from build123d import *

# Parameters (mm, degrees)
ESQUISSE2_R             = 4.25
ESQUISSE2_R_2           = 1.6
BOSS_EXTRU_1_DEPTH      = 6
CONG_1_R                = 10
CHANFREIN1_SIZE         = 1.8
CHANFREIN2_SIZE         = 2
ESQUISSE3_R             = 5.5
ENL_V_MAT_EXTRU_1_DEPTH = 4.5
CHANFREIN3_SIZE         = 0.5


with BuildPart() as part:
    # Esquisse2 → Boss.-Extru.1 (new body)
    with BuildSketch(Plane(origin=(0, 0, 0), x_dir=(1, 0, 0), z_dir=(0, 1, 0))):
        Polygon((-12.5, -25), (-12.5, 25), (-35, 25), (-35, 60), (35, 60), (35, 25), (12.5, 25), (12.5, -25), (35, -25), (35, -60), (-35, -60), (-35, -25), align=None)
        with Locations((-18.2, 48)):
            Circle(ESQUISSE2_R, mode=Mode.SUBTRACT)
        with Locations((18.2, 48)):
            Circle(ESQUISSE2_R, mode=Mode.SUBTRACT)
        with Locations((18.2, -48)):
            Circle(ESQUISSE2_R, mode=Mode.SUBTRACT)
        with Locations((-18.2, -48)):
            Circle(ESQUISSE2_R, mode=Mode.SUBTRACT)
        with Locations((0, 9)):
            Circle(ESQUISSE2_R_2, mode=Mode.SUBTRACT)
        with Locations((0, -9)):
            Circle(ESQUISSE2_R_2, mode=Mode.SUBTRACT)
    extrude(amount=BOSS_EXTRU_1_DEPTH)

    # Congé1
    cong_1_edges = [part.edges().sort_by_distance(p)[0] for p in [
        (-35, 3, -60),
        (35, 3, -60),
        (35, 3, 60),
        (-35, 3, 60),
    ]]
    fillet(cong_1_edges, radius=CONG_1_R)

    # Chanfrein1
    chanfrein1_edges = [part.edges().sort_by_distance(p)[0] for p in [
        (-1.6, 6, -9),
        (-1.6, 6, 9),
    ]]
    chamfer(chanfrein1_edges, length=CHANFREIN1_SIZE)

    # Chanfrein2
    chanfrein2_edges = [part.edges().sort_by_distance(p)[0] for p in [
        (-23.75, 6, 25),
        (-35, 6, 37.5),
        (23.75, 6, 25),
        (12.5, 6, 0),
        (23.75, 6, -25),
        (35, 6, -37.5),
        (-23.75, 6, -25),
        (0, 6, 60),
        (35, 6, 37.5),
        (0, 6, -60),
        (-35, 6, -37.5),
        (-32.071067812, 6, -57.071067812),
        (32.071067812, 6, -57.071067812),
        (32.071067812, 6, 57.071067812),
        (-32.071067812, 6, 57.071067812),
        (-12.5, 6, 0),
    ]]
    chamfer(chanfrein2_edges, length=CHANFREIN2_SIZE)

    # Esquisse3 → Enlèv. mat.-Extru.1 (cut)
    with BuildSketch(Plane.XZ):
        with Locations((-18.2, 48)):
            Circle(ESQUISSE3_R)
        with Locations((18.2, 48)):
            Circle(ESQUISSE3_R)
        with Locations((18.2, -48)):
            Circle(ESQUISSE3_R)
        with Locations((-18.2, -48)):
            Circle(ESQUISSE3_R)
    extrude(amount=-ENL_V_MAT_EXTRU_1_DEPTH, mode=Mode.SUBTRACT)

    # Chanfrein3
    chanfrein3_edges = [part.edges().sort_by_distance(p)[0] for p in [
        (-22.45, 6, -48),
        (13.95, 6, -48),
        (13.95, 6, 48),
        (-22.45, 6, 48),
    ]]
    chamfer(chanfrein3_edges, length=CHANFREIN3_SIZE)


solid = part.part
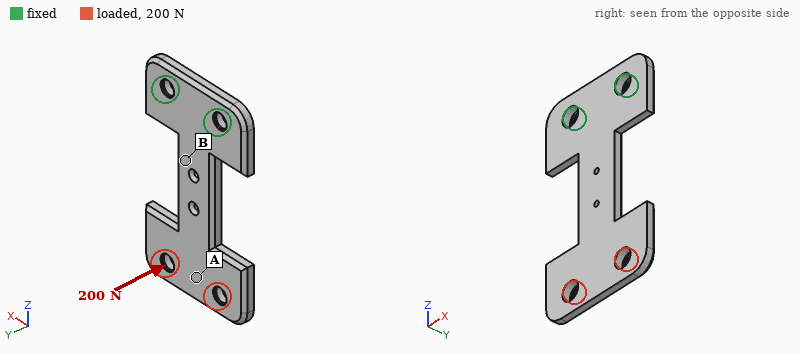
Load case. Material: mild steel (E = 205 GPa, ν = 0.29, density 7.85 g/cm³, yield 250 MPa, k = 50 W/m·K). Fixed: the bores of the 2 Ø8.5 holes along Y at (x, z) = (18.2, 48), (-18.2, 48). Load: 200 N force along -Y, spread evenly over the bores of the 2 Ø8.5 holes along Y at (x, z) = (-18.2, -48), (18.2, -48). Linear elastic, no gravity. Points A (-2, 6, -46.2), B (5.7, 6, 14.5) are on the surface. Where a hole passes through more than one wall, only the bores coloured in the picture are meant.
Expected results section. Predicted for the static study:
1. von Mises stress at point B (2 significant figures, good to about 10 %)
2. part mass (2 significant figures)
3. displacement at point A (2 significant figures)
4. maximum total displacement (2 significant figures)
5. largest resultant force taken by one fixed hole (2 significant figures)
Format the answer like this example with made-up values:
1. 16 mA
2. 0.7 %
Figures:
1. 96 MPa
2. 260 g
3. 0.64 mm
4. 0.78 mm
5. 270 N
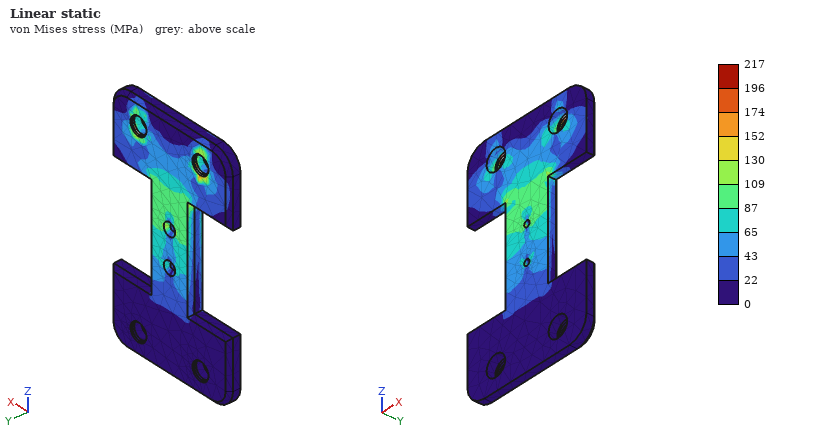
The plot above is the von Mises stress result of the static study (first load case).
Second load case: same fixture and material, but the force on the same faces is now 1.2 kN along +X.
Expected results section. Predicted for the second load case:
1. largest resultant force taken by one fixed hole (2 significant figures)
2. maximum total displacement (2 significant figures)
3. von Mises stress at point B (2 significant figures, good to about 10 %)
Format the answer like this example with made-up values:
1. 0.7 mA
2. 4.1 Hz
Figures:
1. 2.9 kN
2. 0.22 mm
3. 66 MPa
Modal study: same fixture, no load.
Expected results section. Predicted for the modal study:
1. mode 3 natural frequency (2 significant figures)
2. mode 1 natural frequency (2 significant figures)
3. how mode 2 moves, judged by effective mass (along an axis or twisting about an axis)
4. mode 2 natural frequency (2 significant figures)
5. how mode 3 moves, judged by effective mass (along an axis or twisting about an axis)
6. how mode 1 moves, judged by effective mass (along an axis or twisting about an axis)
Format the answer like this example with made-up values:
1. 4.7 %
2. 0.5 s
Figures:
1. 1300 Hz
2. 290 Hz
3. twisting about Z
4. 1000 Hz
5. along X
6. along Y
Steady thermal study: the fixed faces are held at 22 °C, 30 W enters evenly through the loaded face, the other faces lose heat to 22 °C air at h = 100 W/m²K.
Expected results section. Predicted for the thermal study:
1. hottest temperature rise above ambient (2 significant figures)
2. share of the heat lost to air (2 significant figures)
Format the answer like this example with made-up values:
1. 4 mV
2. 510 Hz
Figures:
1. 66 K
2. 96 %
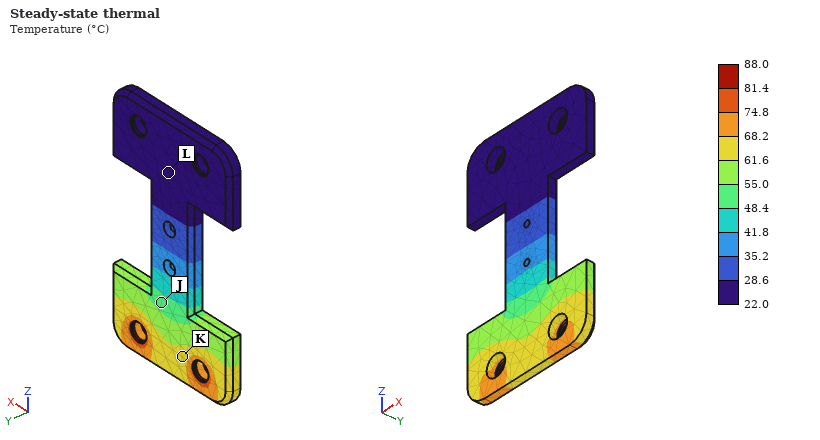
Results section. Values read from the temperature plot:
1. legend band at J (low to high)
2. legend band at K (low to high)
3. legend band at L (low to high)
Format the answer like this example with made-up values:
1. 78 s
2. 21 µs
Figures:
1. 48.4 to 55.0 °C
2. 61.6 to 68.2 °C
3. 22.0 to 28.6 °C
